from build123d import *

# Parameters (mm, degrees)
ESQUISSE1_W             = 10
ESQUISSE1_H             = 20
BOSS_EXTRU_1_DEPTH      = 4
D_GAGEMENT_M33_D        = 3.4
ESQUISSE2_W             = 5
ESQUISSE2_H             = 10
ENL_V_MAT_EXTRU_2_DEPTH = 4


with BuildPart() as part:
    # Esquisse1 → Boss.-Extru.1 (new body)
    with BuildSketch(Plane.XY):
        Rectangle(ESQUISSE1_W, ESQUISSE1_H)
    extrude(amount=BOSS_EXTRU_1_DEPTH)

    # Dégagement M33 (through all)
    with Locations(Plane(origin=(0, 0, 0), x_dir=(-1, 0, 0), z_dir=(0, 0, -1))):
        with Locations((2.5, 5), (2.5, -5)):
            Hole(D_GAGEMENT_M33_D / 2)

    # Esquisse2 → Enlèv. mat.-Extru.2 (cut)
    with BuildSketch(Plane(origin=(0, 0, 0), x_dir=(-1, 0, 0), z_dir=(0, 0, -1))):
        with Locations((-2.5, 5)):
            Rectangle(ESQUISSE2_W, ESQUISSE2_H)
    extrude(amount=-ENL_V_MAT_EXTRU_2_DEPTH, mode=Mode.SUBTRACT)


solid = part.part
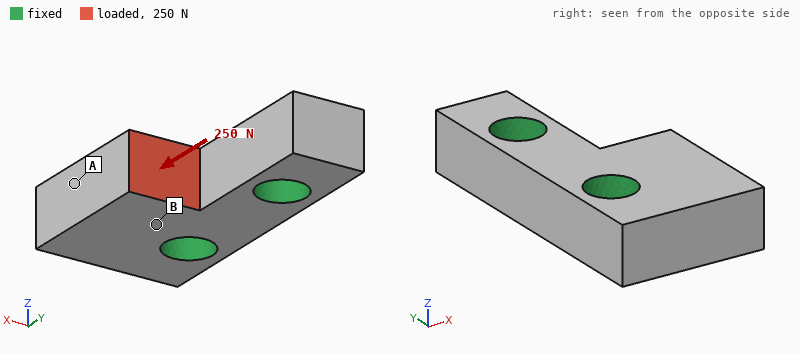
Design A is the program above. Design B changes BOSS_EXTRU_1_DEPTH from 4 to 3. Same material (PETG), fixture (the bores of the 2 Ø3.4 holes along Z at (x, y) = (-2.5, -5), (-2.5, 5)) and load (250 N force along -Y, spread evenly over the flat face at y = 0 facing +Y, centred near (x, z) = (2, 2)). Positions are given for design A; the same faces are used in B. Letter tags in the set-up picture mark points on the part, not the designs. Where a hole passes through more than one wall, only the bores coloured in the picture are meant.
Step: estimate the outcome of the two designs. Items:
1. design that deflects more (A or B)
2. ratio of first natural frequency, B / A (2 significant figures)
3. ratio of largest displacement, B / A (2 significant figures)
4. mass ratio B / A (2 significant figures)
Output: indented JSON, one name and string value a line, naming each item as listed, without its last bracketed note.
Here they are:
{
  "design that deflects more": "B",
  "ratio of first natural frequency, B / A": "0.84",
  "ratio of largest displacement, B / A": "1.3",
  "mass ratio B / A": "0.75"
}
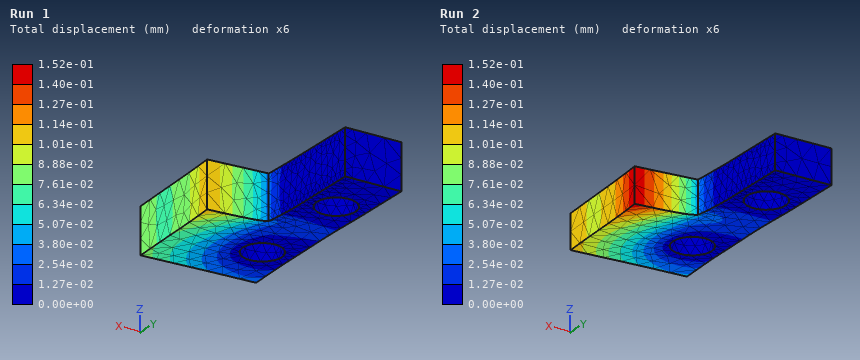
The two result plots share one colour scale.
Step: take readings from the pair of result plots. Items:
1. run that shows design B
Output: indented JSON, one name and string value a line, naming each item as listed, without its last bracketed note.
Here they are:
{
  "run that shows design B": "Run 2"
}
